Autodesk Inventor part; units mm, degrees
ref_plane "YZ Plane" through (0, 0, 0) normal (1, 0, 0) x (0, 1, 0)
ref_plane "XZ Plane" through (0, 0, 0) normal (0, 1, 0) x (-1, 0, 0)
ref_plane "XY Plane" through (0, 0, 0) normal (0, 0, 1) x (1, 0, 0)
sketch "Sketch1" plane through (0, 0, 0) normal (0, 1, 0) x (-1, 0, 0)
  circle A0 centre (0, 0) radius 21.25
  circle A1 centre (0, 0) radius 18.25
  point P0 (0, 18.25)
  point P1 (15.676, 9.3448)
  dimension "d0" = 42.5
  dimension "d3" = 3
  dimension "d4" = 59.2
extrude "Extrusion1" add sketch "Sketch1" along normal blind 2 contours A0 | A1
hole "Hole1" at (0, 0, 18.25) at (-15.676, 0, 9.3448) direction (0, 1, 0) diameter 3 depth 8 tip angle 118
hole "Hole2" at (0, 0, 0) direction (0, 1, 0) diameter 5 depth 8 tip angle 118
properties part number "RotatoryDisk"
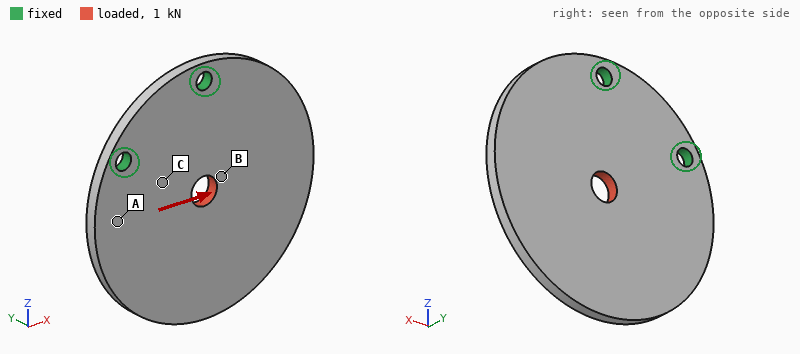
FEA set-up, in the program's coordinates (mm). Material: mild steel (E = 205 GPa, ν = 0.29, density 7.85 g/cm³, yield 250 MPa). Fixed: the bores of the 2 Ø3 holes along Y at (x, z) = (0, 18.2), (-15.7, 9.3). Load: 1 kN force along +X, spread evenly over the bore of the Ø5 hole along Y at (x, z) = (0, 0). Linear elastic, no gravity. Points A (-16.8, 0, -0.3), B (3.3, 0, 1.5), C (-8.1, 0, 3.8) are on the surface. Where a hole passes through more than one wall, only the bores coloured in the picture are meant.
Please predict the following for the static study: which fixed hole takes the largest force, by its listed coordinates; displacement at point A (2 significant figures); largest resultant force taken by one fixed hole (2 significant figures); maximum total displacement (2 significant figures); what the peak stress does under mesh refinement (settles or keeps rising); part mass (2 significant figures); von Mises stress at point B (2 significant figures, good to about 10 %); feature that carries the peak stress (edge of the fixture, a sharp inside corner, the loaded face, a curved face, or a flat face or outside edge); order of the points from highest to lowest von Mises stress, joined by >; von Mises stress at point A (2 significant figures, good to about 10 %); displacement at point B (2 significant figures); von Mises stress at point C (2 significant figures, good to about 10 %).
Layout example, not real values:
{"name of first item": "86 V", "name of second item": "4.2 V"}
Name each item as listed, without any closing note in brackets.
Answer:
{"which fixed hole takes the largest force, by its listed coordinates": "(-15.7, 9.3)", "displacement at point A": "4.4 µm", "largest resultant force taken by one fixed hole": "1.0 kN", "maximum total displacement": "10 µm", "what the peak stress does under mesh refinement": "keeps rising", "part mass": "22 g", "von Mises stress at point B": "29 MPa", "feature that carries the peak stress": "edge of the fixture", "order of the points from highest to lowest von Mises stress, joined by >": "C > B > A", "von Mises stress at point A": "12 MPa", "displacement at point B": "6.1 µm", "von Mises stress at point C": "45 MPa"}
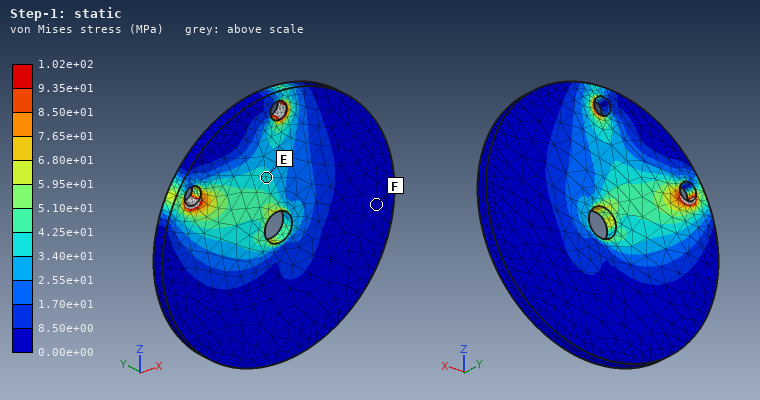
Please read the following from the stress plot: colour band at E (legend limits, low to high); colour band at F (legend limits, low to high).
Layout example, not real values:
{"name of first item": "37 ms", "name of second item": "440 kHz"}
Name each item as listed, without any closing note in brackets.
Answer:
{"colour band at E": "3.40e+01 to 4.25e+01 MPa", "colour band at F": "0.00e+00 to 8.50e+00 MPa"}
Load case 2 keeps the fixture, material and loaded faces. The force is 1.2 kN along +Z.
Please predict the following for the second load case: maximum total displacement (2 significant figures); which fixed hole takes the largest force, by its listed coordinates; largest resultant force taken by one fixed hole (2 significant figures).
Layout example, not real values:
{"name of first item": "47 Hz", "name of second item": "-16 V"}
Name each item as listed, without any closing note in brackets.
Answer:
{"maximum total displacement": "7.1 µm", "which fixed hole takes the largest force, by its listed coordinates": "(0, 18.2)", "largest resultant force taken by one fixed hole": "1.0 kN"}
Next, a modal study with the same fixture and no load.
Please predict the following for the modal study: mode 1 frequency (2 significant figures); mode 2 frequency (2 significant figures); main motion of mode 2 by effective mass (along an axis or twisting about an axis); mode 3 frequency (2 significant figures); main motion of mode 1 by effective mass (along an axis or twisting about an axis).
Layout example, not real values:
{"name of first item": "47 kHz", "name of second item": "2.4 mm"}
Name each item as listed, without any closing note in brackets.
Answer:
{"mode 1 frequency": "1300 Hz", "mode 2 frequency": "3100 Hz", "main motion of mode 2 by effective mass": "twisting about Z", "mode 3 frequency": "6600 Hz", "main motion of mode 1 by effective mass": "along Y"}
